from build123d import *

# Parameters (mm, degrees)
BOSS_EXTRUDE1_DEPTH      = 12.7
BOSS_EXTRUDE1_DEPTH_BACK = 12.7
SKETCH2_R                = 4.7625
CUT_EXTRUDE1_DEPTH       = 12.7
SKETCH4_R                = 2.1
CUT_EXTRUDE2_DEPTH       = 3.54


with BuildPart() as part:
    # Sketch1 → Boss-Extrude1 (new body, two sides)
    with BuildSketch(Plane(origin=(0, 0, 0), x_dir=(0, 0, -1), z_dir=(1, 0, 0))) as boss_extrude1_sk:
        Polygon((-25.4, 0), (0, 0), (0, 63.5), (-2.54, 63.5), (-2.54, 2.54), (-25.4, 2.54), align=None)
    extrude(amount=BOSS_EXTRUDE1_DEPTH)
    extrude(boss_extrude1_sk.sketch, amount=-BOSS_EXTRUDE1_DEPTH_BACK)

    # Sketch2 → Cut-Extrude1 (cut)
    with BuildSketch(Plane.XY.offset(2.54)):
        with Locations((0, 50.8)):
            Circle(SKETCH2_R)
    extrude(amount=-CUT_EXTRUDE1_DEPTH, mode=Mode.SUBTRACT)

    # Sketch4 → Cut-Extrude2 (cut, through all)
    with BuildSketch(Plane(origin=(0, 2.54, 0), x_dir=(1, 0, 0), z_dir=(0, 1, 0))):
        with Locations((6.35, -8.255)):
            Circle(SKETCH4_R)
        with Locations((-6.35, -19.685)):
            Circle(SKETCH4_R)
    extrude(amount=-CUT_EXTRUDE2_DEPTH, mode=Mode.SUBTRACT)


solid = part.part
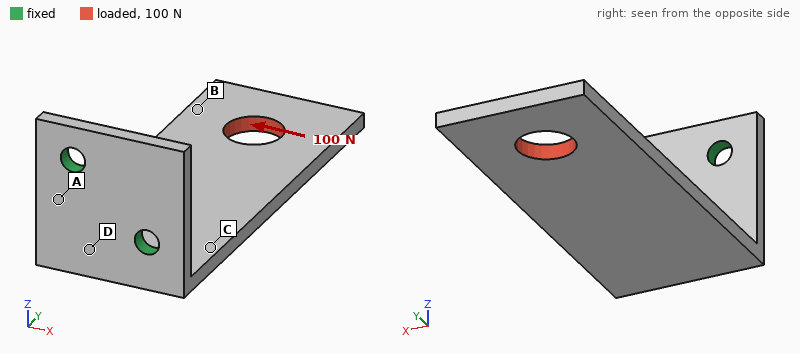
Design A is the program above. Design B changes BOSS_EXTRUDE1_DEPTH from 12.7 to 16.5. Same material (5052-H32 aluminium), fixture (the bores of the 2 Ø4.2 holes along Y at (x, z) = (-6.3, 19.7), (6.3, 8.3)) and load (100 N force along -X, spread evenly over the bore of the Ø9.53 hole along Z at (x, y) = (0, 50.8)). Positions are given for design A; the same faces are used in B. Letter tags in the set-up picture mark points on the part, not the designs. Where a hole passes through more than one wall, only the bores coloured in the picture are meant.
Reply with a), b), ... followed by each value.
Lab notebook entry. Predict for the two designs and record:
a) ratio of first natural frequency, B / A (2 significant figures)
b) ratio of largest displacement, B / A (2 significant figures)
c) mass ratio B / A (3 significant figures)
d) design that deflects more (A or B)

a) 1.00
b) 0.83
c) 1.16
d) A
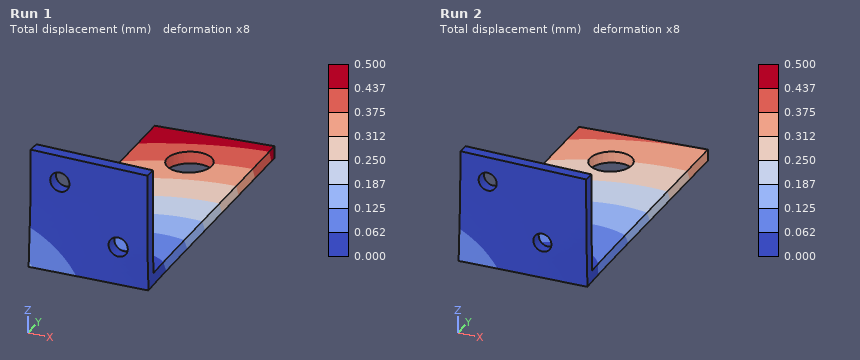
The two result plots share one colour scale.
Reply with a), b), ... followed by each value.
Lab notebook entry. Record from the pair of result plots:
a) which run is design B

a) Run 2
